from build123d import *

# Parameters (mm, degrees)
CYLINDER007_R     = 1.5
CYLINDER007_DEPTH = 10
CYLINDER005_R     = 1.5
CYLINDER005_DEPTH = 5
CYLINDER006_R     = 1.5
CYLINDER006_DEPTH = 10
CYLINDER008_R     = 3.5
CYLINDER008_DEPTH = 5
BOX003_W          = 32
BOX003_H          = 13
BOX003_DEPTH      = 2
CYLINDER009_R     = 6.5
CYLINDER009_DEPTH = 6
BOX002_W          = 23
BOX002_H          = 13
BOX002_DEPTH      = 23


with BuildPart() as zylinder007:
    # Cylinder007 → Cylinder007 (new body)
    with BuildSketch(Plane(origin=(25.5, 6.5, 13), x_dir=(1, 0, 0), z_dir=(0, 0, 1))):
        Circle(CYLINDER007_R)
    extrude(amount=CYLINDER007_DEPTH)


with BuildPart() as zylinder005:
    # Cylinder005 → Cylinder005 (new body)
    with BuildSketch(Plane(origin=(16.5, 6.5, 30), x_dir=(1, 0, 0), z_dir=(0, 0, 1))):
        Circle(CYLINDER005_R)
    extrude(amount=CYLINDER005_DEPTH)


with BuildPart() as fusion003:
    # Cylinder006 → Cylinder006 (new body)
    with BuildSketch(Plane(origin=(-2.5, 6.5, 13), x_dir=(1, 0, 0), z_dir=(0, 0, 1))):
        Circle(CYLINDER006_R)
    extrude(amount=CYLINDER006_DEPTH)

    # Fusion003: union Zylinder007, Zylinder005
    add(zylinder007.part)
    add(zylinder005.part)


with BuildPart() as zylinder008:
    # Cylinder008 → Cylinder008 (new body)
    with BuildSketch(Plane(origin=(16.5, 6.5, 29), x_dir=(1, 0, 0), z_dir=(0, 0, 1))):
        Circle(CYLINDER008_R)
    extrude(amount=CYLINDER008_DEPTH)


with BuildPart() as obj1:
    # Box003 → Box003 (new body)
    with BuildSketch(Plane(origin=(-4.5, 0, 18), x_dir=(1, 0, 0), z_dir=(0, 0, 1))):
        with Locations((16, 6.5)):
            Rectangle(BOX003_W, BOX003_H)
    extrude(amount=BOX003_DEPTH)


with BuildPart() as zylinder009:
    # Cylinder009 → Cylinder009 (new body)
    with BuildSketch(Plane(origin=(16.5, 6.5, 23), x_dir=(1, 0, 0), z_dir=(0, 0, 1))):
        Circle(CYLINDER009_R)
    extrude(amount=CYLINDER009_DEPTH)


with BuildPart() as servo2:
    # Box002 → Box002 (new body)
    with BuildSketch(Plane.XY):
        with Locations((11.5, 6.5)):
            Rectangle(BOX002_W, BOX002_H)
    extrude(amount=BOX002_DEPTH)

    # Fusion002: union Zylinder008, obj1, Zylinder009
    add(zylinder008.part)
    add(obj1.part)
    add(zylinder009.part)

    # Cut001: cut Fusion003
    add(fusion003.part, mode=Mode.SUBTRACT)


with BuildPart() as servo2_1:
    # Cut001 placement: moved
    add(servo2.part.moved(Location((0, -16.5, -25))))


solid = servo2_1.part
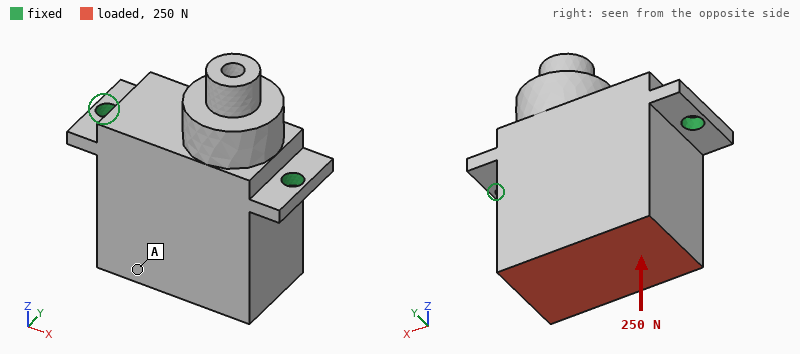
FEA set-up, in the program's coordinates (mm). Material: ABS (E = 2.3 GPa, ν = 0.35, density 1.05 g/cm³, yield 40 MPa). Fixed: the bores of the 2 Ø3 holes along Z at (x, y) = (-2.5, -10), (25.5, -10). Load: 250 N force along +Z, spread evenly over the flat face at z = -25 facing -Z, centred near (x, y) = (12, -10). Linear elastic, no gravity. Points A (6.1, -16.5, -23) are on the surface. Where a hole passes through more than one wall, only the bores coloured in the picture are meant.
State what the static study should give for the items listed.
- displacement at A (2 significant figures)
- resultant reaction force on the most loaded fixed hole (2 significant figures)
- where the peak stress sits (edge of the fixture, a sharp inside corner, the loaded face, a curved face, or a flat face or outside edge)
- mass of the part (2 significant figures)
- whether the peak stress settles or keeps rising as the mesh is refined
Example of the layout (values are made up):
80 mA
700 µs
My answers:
46 µm
130 N
edge of the fixture
8.4 g
keeps rising
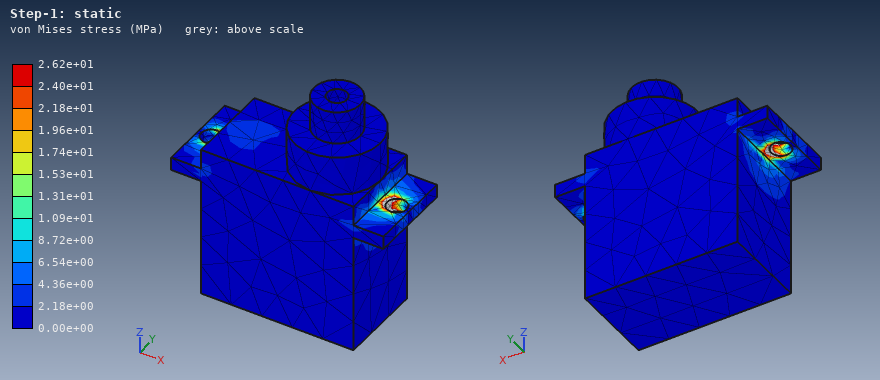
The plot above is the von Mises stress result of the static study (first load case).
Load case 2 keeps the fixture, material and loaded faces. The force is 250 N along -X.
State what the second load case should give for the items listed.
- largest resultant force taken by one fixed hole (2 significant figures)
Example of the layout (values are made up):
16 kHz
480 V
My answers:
230 N
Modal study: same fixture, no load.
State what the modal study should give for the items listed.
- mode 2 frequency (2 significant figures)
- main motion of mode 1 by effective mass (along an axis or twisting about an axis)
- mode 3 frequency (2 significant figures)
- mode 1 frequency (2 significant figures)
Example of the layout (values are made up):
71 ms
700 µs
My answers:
4200 Hz
along Y
4300 Hz
930 Hz
